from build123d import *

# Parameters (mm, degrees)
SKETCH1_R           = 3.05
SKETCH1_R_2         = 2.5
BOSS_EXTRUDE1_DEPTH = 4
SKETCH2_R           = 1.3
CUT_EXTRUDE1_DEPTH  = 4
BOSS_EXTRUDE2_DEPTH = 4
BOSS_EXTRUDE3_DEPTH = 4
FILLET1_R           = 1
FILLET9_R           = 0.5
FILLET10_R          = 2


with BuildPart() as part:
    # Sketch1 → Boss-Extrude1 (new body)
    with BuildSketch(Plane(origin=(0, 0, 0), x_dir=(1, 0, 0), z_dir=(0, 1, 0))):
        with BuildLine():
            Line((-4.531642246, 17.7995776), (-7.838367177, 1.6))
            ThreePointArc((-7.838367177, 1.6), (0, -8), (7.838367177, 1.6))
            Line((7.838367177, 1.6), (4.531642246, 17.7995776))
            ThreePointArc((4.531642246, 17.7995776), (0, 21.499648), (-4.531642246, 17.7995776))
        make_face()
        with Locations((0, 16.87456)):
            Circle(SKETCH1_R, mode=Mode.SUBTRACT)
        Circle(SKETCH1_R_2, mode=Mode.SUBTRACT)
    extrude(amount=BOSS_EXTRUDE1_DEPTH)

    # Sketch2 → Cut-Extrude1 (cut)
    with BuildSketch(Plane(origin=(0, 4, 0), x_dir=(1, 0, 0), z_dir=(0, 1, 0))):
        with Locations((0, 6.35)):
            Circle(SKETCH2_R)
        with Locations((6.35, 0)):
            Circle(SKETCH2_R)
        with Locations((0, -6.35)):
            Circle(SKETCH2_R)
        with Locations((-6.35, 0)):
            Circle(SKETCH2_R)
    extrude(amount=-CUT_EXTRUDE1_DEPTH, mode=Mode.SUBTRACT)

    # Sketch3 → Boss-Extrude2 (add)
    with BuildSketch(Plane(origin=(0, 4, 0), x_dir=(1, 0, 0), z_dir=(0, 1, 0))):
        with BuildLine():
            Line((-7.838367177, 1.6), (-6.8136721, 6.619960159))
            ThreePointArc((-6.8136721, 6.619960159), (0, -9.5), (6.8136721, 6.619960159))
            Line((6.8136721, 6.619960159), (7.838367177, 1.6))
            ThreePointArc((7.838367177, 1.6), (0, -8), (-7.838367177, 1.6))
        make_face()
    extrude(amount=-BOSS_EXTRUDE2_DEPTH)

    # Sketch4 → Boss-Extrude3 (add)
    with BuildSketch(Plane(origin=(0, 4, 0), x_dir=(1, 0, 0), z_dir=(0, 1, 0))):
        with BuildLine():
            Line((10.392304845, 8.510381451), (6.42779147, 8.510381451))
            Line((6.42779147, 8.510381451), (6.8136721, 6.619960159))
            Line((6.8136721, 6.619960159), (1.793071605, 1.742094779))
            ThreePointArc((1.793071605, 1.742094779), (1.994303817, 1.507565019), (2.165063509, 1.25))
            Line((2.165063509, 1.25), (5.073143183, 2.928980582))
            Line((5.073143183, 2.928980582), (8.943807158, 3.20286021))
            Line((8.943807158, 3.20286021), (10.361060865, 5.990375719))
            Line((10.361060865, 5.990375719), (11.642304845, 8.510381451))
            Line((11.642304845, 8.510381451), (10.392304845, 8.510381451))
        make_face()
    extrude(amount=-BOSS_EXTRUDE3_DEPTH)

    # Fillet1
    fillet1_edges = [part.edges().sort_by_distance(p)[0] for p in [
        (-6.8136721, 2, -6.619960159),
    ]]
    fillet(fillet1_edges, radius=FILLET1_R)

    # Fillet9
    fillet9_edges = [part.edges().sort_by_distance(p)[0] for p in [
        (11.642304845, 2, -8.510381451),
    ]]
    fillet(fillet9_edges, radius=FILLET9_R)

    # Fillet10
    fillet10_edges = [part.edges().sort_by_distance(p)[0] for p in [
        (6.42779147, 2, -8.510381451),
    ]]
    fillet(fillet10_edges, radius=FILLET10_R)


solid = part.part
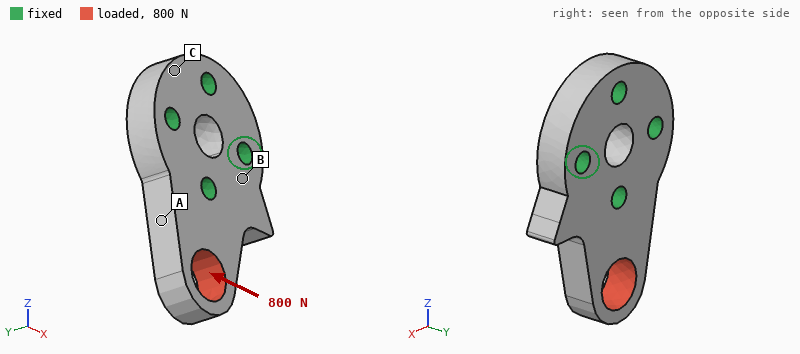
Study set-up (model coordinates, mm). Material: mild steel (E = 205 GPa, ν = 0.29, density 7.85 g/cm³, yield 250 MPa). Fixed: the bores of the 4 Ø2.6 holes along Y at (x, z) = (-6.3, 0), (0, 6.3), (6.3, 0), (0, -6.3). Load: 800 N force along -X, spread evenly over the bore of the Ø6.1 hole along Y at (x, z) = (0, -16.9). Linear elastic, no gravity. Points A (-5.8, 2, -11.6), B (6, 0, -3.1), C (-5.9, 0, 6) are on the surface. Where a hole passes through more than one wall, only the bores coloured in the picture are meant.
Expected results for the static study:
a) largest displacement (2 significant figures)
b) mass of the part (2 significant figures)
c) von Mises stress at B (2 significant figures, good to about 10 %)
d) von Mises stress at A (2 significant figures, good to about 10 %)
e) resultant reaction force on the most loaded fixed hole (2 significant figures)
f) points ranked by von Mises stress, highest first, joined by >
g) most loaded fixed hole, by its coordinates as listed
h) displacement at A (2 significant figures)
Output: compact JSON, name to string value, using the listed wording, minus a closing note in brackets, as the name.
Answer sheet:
{"largest displacement": "16 µm", "mass of the part": "11 g", "von Mises stress at B": "31 MPa", "von Mises stress at A": "74 MPa", "resultant reaction force on the most loaded fixed hole": "780 N", "points ranked by von Mises stress, highest first, joined by >": "A > B > C", "most loaded fixed hole, by its coordinates as listed": "(0, -6.3)", "displacement at A": "3.3 µm"}
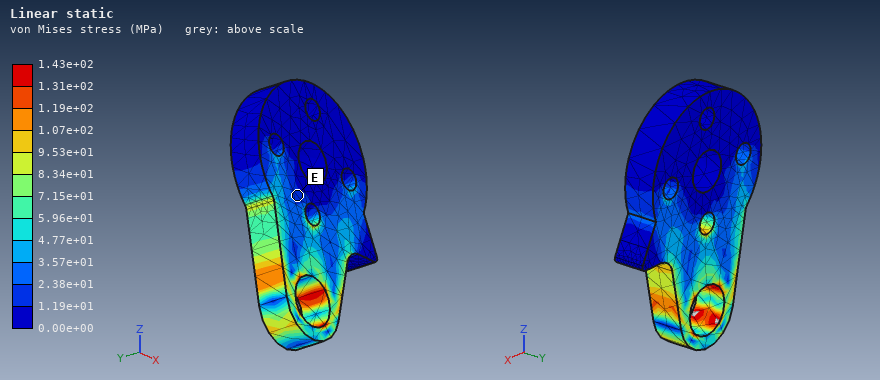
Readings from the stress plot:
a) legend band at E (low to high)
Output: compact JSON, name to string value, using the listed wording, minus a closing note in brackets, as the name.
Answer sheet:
{"legend band at E": "1.19e+01 to 2.38e+01 MPa"}
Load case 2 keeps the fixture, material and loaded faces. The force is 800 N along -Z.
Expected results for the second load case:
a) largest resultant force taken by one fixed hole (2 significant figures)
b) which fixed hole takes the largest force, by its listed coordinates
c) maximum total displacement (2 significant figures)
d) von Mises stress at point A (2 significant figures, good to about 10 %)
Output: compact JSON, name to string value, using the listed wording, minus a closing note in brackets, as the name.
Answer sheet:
{"largest resultant force taken by one fixed hole": "500 N", "which fixed hole takes the largest force, by its listed coordinates": "(0, -6.3)", "maximum total displacement": "3.1 µm", "von Mises stress at point A": "25 MPa"}
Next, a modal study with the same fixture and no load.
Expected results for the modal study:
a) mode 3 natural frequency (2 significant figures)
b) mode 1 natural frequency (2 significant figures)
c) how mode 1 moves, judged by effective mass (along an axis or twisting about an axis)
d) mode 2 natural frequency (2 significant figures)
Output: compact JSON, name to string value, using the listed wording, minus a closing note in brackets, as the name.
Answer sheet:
{"mode 3 natural frequency": "40 kHz", "mode 1 natural frequency": "21 kHz", "how mode 1 moves, judged by effective mass": "along Y", "mode 2 natural frequency": "35 kHz"}
